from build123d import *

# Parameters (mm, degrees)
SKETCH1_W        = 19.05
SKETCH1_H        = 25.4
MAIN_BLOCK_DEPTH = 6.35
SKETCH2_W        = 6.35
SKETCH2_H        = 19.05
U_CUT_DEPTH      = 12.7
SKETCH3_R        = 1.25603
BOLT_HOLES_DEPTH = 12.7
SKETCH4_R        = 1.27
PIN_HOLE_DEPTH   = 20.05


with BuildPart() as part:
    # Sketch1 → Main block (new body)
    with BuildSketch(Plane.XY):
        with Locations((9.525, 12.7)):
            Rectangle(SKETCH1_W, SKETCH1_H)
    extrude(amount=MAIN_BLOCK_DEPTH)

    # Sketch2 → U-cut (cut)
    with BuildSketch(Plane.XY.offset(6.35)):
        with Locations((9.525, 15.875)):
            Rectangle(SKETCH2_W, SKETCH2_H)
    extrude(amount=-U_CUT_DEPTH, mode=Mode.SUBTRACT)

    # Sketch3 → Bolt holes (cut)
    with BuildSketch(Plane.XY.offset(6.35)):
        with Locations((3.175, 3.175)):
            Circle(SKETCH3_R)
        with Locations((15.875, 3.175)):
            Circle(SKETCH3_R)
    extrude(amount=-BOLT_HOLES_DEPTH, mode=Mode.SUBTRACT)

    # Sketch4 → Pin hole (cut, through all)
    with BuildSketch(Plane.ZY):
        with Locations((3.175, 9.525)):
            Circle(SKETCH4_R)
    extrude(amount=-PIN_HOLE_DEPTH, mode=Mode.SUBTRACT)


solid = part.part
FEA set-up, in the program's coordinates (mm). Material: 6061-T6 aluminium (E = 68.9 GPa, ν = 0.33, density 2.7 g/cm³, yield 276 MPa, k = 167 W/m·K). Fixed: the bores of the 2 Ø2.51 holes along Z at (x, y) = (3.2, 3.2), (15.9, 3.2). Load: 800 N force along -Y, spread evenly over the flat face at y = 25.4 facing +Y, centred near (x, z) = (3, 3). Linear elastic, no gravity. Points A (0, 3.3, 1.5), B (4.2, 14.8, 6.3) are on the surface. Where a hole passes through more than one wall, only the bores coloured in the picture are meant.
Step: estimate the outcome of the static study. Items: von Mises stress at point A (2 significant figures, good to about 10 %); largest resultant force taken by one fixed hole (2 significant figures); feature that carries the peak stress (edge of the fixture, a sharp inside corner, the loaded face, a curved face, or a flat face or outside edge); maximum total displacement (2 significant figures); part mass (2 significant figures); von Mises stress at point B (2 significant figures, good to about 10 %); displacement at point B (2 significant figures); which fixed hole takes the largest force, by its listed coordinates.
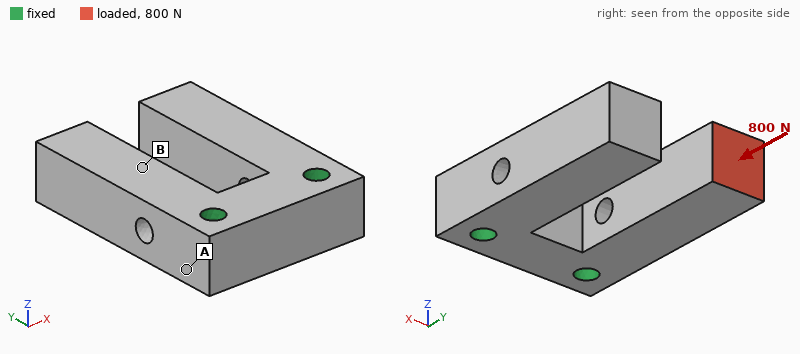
9.6 MPa
780 N
a curved face
7.7 µm
5.9 g
22 MPa
4.1 µm
(3.2, 3.2)
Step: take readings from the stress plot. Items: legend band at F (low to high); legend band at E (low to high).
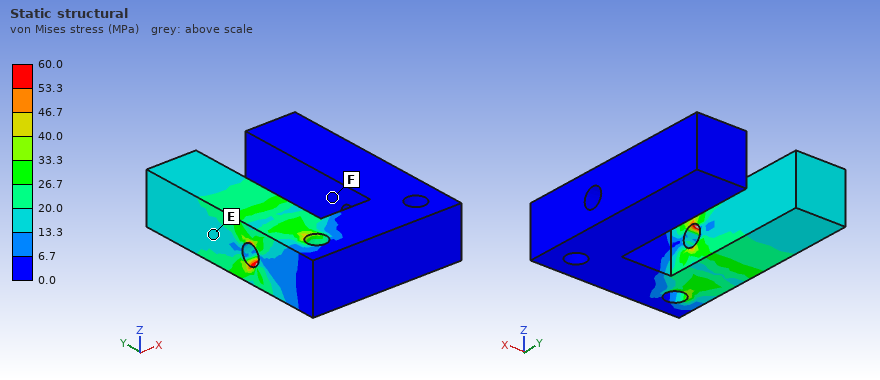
0.0 to 6.7 MPa
13.3 to 20.0 MPa
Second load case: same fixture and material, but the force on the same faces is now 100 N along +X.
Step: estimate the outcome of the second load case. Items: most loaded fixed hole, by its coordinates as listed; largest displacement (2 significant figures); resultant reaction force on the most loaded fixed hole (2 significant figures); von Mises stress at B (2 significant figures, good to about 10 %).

(15.9, 3.2)
50 µm
130 N
12 MPa
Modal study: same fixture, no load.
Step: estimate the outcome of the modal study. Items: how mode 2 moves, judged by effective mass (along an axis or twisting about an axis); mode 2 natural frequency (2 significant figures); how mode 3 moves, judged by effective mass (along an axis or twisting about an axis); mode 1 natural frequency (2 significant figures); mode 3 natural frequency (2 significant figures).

along X
9400 Hz
along Z
9000 Hz
10 kHz
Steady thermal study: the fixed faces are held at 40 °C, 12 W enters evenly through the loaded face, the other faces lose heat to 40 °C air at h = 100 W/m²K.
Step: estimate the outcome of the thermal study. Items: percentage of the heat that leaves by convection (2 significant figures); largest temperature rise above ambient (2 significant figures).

9.5 %
39 K
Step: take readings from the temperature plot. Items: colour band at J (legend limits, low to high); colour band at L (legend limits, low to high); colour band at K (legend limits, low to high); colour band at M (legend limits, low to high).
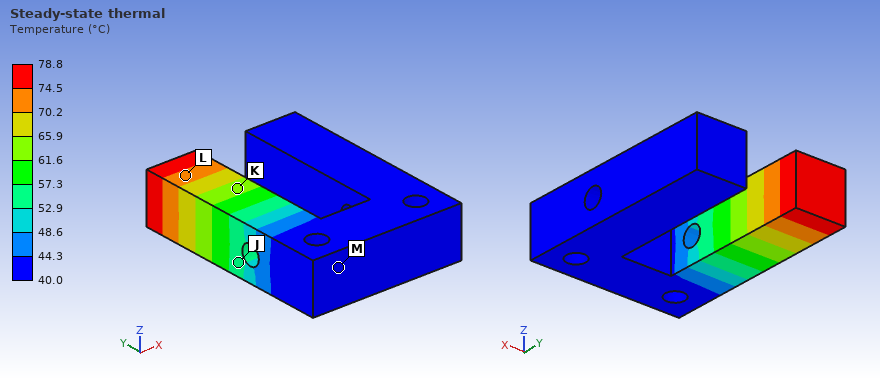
52.9 to 57.3 °C
70.2 to 74.5 °C
61.6 to 65.9 °C
40.0 to 44.3 °C
